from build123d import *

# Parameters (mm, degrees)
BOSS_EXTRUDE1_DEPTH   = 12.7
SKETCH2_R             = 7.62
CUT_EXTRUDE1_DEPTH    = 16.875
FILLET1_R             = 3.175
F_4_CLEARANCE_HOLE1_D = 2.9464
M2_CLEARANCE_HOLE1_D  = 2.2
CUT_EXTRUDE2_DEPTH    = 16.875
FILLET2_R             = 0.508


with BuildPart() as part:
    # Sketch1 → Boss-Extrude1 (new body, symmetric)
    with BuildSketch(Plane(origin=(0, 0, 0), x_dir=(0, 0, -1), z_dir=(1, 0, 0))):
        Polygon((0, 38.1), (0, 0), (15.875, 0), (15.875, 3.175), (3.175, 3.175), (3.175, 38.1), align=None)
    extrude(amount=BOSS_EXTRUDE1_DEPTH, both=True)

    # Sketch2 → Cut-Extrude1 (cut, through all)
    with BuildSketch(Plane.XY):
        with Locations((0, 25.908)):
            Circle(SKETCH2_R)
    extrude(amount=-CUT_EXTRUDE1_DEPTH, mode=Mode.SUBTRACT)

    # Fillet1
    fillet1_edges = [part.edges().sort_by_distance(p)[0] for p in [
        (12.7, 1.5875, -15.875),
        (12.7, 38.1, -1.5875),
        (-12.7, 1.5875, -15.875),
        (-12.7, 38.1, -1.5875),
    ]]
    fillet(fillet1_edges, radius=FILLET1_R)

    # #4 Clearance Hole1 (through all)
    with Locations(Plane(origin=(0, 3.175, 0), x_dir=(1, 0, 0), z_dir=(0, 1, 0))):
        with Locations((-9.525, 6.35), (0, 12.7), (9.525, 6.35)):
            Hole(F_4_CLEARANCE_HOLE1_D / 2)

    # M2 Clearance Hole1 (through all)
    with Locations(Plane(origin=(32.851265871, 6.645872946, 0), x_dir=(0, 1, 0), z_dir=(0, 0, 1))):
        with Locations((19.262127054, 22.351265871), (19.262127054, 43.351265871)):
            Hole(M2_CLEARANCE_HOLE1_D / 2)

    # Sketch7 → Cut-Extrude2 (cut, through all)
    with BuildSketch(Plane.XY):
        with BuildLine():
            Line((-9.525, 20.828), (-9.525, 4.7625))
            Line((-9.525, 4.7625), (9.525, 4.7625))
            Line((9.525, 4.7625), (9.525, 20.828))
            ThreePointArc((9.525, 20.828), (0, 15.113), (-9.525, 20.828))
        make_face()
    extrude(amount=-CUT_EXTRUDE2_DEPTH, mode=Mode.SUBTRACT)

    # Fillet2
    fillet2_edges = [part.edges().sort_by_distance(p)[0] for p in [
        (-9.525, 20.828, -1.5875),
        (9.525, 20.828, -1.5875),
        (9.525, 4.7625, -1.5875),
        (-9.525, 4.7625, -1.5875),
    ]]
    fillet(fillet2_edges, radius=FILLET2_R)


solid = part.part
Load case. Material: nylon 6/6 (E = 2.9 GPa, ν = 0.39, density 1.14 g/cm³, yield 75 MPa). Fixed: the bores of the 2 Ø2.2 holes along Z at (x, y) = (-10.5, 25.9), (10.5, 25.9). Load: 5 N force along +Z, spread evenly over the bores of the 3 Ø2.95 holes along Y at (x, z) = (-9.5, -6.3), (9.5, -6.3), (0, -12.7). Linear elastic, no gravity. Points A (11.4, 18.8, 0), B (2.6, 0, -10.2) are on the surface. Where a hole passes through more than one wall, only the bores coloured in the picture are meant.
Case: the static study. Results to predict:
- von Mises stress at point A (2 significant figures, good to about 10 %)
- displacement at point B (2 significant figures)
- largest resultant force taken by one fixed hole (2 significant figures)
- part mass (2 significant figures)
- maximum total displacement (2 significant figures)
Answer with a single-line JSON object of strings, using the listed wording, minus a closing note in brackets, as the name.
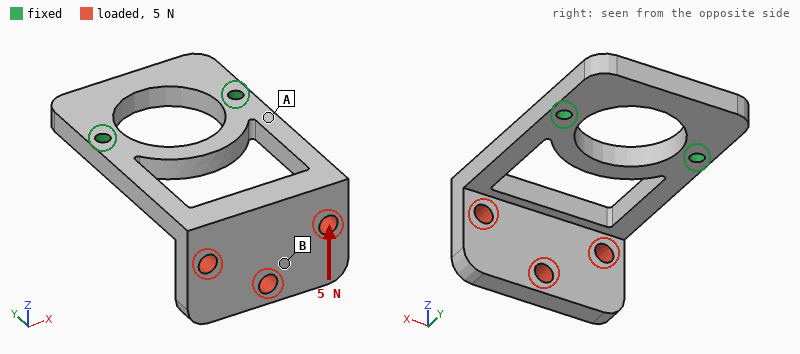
{"von Mises stress at point A": "7.5 MPa", "displacement at point B": "0.47 mm", "largest resultant force taken by one fixed hole": "2.5 N", "part mass": "3.1 g", "maximum total displacement": "0.55 mm"}
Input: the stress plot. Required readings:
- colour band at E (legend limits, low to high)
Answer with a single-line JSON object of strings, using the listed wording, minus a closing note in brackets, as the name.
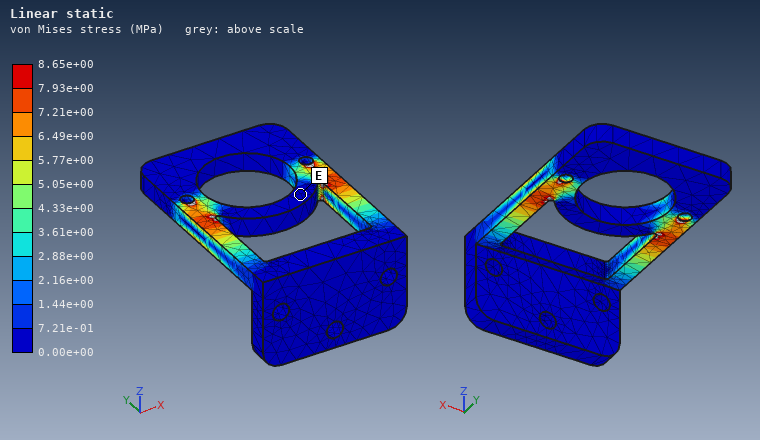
{"colour band at E": "0.00e+00 to 7.21e-01 MPa"}
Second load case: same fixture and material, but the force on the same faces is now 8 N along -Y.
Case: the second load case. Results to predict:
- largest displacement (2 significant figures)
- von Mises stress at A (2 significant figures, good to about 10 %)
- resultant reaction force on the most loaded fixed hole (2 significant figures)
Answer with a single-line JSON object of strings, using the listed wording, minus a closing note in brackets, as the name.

{"largest displacement": "0.48 mm", "von Mises stress at A": "4.5 MPa", "resultant reaction force on the most loaded fixed hole": "4.0 N"}
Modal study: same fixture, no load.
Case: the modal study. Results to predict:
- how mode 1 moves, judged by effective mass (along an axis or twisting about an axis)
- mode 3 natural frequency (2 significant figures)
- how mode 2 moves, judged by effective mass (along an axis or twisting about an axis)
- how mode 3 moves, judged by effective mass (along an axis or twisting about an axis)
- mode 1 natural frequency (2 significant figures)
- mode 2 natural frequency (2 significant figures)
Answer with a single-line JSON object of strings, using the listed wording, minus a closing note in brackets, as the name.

{"how mode 1 moves, judged by effective mass": "along Z", "mode 3 natural frequency": "1400 Hz", "how mode 2 moves, judged by effective mass": "along X", "how mode 3 moves, judged by effective mass": "along X", "mode 1 natural frequency": "420 Hz", "mode 2 natural frequency": "840 Hz"}
